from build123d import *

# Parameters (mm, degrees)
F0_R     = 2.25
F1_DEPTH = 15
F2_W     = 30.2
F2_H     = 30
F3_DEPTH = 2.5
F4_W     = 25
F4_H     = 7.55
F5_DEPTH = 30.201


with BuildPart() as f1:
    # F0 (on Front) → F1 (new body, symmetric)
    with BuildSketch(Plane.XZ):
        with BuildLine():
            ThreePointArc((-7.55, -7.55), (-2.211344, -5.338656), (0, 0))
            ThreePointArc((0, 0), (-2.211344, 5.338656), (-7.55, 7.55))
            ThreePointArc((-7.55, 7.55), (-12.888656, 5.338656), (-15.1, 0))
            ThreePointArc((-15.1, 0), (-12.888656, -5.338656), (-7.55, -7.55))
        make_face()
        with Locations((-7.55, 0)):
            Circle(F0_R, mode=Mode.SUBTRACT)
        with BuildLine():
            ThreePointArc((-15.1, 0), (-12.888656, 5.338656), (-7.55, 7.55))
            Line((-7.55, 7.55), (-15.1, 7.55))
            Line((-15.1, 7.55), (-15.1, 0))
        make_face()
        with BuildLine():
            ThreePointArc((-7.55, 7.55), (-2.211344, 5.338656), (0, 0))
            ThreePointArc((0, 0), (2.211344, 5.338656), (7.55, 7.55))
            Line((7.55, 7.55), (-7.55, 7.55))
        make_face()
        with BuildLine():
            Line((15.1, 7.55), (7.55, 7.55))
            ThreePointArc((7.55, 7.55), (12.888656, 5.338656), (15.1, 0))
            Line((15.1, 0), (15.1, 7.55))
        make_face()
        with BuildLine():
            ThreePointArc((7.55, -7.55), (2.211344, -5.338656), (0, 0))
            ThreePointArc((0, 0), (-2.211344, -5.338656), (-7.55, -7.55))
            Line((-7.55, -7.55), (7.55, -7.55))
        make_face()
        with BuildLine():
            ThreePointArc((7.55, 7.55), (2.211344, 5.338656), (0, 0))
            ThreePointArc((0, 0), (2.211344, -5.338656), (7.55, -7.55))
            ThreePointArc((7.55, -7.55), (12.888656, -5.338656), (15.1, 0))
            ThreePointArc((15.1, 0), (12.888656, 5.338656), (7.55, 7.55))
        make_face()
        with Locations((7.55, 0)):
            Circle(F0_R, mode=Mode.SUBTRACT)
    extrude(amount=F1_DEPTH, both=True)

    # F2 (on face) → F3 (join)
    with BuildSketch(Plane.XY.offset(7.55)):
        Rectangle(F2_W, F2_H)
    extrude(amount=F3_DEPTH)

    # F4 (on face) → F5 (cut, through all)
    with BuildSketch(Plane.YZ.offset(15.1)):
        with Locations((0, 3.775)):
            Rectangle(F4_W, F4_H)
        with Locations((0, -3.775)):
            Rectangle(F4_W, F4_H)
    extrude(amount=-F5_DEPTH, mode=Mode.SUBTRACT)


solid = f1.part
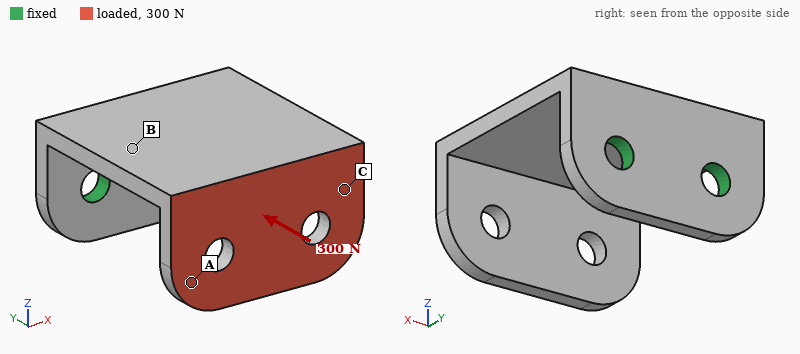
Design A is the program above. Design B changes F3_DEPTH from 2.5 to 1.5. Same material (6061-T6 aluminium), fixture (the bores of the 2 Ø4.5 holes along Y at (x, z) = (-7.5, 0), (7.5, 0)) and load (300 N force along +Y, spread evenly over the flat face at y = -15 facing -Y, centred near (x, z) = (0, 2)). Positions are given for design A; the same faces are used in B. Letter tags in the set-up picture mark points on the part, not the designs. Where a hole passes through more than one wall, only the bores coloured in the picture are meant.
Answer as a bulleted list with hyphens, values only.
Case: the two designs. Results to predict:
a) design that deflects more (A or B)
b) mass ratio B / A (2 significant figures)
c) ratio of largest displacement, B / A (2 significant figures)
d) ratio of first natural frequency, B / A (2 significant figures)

- B
- 0.79
- 3.8
- 0.63
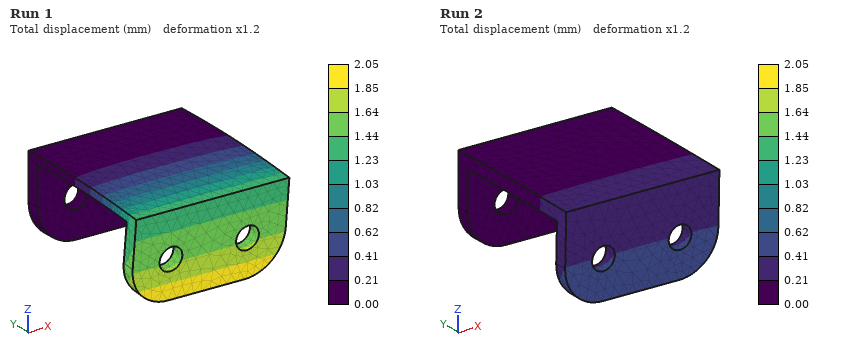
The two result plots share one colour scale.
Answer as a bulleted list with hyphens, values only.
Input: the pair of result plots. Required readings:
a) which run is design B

- Run 1
